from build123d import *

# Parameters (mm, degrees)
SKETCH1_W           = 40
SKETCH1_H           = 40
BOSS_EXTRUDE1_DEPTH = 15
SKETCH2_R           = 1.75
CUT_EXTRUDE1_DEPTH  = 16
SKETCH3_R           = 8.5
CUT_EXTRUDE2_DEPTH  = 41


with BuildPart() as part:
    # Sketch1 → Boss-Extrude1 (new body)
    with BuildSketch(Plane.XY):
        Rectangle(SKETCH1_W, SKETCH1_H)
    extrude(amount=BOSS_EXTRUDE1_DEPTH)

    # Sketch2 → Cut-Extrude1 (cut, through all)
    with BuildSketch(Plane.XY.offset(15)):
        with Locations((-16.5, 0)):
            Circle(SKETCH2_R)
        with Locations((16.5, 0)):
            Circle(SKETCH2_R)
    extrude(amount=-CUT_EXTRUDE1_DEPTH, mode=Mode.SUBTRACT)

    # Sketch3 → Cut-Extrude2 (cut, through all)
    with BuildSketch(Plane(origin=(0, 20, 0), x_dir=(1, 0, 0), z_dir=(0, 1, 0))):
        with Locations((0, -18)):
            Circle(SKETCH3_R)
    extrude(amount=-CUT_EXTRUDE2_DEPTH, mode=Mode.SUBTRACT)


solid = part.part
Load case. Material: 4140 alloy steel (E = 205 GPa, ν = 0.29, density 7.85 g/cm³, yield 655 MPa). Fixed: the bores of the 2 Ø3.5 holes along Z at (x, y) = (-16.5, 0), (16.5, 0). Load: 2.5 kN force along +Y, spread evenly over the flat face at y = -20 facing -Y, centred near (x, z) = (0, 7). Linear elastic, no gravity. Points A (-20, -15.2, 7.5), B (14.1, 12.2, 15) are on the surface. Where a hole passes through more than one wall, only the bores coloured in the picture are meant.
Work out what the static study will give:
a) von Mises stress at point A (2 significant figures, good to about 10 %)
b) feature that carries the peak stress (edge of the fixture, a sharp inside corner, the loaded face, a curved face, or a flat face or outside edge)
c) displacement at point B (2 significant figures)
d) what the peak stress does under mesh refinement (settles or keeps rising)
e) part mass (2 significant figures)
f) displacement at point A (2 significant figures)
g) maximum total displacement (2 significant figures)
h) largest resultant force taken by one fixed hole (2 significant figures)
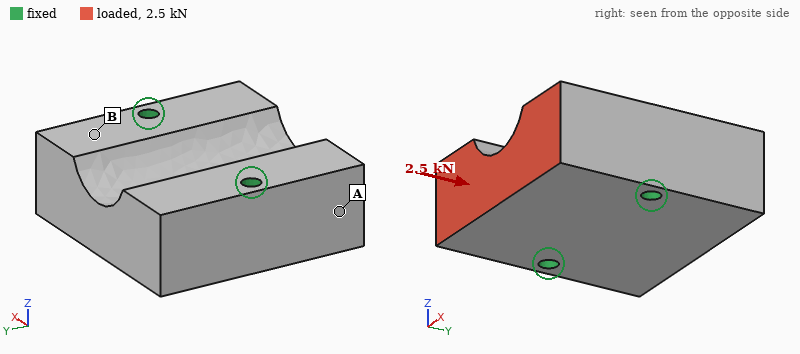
4.9 MPa
edge of the fixture
0.14 µm
keeps rising
170 g
0.42 µm
0.79 µm
1.3 kN
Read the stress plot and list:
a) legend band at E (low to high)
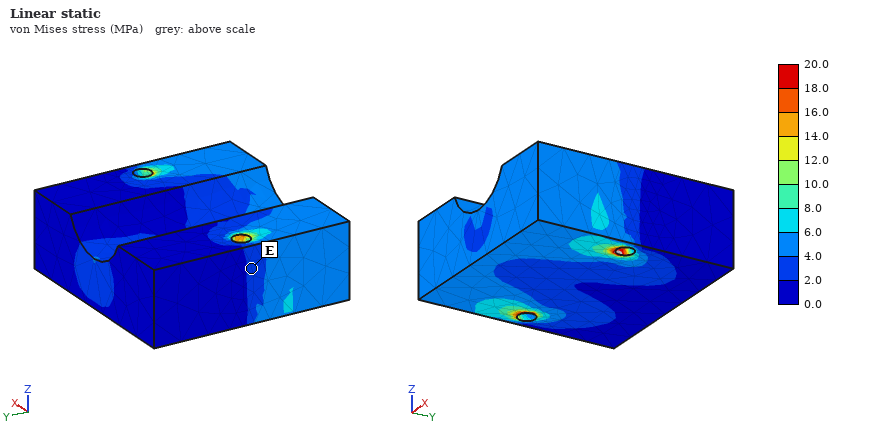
2.0 to 4.0 MPa
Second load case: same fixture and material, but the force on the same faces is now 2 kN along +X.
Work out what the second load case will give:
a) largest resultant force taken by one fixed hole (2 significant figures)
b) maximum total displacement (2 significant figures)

1.5 kN
2.2 µm
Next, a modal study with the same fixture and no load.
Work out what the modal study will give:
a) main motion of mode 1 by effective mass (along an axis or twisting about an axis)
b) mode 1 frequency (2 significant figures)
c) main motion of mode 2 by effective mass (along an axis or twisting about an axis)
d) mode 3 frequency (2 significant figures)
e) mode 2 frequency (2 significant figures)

twisting about X
17 kHz
along Z
25 kHz
20 kHz
